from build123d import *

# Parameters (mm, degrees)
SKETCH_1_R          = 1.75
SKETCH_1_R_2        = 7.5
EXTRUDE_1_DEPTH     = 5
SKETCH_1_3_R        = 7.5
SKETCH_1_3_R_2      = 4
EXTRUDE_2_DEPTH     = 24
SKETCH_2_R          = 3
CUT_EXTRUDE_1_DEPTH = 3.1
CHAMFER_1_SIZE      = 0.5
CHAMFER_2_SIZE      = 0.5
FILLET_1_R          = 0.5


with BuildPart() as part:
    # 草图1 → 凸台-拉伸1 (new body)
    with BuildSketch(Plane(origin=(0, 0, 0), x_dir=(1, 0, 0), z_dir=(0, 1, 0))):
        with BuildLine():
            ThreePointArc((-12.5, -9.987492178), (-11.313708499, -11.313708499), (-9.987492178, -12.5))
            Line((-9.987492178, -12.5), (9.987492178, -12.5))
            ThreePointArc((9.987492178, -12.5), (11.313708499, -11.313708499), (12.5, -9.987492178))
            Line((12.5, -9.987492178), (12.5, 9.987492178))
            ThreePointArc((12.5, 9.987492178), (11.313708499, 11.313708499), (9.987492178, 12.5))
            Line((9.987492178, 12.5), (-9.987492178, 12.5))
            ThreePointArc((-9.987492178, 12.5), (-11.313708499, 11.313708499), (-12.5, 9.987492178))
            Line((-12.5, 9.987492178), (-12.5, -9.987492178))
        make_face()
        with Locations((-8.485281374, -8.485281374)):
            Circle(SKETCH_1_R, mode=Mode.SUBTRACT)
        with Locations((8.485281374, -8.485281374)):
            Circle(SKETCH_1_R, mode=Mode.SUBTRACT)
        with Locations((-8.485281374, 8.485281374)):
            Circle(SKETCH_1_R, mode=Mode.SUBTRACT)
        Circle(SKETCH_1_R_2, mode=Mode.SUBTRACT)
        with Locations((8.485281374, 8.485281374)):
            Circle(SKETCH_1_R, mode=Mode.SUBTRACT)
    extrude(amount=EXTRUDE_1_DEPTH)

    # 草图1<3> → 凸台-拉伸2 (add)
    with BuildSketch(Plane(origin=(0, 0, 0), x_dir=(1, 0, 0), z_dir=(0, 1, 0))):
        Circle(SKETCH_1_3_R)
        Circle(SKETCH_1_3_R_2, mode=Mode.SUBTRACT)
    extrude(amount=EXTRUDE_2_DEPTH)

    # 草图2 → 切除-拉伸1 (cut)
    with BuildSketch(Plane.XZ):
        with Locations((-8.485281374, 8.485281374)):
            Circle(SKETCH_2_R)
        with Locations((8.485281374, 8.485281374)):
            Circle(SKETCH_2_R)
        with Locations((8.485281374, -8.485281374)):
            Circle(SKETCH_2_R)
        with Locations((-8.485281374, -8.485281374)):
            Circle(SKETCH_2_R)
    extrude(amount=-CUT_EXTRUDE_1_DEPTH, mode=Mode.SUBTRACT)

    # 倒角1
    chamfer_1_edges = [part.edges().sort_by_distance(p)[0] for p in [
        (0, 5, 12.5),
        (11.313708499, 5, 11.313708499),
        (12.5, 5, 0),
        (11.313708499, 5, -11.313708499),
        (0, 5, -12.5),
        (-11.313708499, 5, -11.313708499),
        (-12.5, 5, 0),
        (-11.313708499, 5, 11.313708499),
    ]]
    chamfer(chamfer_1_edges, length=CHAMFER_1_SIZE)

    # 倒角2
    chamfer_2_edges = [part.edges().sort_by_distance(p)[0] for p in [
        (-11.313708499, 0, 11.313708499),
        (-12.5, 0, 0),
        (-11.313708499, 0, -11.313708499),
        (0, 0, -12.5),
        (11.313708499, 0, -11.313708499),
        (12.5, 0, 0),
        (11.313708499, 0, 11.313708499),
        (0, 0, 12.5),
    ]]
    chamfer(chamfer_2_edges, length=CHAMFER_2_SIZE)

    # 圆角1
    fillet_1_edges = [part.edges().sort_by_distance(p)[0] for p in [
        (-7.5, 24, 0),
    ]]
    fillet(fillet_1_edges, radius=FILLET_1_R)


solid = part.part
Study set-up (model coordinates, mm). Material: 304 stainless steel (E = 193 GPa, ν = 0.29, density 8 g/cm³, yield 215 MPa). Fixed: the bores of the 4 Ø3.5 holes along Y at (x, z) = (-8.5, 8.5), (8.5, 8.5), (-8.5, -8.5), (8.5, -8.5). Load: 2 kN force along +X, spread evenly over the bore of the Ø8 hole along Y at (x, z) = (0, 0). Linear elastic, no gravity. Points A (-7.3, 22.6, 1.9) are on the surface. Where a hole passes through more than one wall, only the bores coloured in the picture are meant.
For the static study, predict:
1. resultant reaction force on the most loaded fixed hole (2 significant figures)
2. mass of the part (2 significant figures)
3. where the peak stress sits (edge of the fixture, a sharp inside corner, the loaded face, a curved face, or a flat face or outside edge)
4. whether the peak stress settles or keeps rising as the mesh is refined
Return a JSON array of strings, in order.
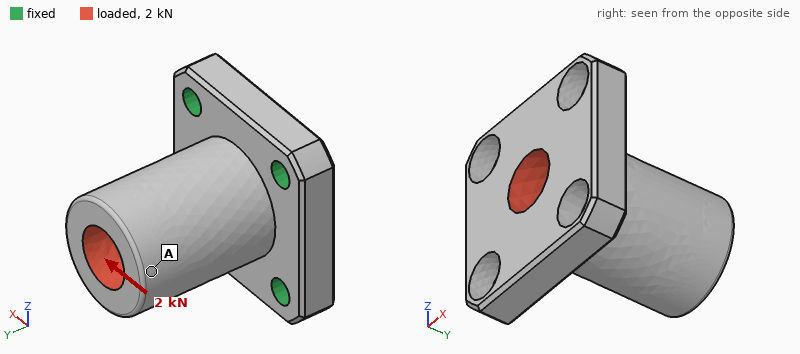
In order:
["710 N", "38 g", "edge of the fixture", "keeps rising"]
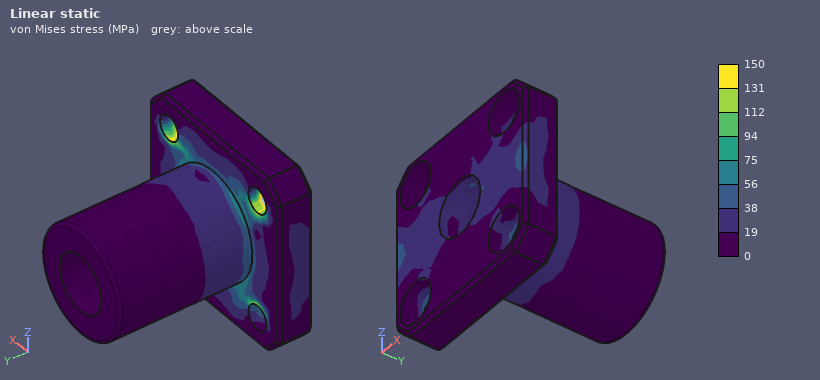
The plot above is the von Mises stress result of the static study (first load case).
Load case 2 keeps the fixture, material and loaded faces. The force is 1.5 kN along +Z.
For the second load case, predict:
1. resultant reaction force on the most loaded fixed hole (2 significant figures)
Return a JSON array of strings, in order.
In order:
["530 N"]
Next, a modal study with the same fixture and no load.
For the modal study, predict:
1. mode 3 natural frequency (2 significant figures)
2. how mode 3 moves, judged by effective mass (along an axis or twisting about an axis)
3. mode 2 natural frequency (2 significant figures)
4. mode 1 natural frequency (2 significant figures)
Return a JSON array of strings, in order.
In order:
["26 kHz", "along Y", "14 kHz", "14 kHz"]
